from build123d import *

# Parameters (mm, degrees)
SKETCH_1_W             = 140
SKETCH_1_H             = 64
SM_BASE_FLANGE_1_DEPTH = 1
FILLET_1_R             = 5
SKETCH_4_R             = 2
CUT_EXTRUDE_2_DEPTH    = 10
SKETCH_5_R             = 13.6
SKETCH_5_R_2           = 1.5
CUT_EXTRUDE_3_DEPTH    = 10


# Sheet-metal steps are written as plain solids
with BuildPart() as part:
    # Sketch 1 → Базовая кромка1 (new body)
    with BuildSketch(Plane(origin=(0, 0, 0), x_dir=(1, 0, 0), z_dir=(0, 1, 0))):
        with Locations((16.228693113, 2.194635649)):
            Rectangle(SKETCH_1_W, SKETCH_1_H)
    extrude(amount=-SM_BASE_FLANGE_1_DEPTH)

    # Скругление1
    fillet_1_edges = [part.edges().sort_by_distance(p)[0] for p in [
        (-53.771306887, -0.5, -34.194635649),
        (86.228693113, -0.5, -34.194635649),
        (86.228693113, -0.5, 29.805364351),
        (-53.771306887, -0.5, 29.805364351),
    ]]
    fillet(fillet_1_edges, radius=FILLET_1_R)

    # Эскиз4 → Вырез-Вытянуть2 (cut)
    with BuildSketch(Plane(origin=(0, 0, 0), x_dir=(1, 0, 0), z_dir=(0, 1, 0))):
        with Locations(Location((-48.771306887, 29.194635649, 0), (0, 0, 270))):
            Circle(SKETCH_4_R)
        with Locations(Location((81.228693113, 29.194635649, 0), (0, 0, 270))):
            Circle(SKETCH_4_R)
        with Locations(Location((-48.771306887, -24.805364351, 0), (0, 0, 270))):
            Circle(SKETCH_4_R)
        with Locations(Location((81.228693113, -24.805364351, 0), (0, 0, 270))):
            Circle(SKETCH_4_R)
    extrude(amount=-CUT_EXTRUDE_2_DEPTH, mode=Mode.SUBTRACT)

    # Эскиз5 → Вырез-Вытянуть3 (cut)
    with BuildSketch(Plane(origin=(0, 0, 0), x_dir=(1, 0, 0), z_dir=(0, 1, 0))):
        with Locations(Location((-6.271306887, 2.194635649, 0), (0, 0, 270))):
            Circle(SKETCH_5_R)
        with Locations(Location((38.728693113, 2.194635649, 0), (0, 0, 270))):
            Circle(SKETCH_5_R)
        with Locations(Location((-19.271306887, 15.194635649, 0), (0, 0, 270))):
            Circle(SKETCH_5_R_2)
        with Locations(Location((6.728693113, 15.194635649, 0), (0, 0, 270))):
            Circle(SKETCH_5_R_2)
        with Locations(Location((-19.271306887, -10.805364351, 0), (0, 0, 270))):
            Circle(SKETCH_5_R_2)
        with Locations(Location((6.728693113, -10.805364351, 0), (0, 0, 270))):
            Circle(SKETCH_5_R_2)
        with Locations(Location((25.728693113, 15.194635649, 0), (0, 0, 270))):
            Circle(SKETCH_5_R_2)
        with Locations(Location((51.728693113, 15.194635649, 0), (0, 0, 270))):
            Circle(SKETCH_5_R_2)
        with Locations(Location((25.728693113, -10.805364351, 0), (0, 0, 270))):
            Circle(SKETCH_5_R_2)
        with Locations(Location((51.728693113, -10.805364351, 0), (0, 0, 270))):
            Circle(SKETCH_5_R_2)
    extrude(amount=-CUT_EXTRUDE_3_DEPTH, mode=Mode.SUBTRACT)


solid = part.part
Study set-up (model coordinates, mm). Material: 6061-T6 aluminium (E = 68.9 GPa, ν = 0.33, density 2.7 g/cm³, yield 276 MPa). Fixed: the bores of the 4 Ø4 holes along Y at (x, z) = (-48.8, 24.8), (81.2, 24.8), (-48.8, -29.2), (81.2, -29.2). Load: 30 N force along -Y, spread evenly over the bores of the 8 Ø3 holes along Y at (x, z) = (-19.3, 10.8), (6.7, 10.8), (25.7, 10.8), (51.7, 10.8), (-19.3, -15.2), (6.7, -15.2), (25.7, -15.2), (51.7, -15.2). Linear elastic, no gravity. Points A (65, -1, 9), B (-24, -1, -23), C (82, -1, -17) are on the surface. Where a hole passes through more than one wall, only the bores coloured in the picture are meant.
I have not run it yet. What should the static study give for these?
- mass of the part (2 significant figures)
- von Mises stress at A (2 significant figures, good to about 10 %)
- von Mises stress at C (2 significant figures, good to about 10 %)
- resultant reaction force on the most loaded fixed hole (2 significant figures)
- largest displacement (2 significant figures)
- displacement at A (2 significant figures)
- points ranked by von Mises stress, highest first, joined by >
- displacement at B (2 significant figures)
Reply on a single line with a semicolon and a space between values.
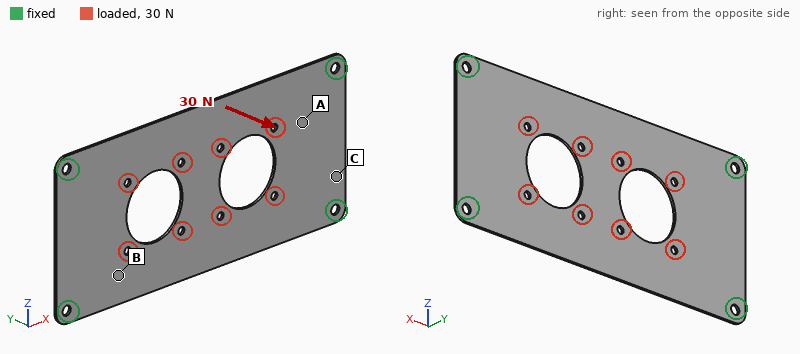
21 g; 16 MPa; 25 MPa; 7.5 N; 0.93 mm; 0.22 mm; C > A > B; 0.36 mm
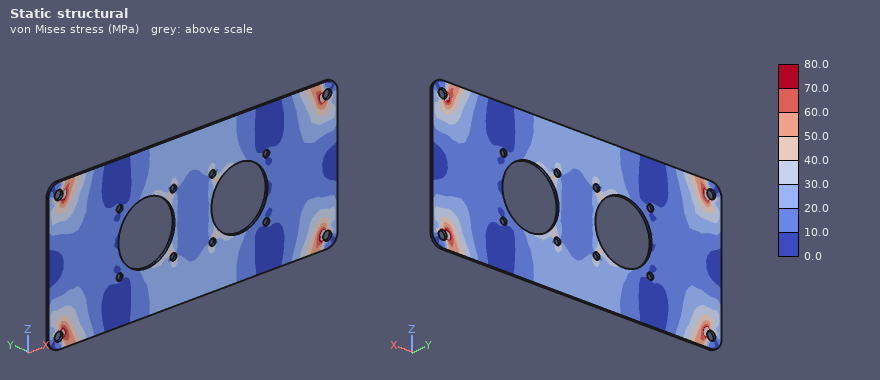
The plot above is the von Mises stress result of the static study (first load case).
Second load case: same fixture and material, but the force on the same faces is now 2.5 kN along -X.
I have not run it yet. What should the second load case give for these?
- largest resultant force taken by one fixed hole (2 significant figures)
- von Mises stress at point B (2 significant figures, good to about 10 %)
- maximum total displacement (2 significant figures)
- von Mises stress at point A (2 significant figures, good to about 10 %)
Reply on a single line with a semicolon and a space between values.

650 N; 28 MPa; 29 µm; 14 MPa
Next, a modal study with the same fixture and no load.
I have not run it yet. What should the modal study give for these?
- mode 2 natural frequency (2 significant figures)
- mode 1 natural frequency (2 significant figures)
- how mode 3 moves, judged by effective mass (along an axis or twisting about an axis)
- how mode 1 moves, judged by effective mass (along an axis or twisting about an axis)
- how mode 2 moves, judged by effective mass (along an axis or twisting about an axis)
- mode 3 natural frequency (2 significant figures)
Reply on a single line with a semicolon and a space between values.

490 Hz; 290 Hz; twisting about Z; along Y; twisting about X; 780 Hz
